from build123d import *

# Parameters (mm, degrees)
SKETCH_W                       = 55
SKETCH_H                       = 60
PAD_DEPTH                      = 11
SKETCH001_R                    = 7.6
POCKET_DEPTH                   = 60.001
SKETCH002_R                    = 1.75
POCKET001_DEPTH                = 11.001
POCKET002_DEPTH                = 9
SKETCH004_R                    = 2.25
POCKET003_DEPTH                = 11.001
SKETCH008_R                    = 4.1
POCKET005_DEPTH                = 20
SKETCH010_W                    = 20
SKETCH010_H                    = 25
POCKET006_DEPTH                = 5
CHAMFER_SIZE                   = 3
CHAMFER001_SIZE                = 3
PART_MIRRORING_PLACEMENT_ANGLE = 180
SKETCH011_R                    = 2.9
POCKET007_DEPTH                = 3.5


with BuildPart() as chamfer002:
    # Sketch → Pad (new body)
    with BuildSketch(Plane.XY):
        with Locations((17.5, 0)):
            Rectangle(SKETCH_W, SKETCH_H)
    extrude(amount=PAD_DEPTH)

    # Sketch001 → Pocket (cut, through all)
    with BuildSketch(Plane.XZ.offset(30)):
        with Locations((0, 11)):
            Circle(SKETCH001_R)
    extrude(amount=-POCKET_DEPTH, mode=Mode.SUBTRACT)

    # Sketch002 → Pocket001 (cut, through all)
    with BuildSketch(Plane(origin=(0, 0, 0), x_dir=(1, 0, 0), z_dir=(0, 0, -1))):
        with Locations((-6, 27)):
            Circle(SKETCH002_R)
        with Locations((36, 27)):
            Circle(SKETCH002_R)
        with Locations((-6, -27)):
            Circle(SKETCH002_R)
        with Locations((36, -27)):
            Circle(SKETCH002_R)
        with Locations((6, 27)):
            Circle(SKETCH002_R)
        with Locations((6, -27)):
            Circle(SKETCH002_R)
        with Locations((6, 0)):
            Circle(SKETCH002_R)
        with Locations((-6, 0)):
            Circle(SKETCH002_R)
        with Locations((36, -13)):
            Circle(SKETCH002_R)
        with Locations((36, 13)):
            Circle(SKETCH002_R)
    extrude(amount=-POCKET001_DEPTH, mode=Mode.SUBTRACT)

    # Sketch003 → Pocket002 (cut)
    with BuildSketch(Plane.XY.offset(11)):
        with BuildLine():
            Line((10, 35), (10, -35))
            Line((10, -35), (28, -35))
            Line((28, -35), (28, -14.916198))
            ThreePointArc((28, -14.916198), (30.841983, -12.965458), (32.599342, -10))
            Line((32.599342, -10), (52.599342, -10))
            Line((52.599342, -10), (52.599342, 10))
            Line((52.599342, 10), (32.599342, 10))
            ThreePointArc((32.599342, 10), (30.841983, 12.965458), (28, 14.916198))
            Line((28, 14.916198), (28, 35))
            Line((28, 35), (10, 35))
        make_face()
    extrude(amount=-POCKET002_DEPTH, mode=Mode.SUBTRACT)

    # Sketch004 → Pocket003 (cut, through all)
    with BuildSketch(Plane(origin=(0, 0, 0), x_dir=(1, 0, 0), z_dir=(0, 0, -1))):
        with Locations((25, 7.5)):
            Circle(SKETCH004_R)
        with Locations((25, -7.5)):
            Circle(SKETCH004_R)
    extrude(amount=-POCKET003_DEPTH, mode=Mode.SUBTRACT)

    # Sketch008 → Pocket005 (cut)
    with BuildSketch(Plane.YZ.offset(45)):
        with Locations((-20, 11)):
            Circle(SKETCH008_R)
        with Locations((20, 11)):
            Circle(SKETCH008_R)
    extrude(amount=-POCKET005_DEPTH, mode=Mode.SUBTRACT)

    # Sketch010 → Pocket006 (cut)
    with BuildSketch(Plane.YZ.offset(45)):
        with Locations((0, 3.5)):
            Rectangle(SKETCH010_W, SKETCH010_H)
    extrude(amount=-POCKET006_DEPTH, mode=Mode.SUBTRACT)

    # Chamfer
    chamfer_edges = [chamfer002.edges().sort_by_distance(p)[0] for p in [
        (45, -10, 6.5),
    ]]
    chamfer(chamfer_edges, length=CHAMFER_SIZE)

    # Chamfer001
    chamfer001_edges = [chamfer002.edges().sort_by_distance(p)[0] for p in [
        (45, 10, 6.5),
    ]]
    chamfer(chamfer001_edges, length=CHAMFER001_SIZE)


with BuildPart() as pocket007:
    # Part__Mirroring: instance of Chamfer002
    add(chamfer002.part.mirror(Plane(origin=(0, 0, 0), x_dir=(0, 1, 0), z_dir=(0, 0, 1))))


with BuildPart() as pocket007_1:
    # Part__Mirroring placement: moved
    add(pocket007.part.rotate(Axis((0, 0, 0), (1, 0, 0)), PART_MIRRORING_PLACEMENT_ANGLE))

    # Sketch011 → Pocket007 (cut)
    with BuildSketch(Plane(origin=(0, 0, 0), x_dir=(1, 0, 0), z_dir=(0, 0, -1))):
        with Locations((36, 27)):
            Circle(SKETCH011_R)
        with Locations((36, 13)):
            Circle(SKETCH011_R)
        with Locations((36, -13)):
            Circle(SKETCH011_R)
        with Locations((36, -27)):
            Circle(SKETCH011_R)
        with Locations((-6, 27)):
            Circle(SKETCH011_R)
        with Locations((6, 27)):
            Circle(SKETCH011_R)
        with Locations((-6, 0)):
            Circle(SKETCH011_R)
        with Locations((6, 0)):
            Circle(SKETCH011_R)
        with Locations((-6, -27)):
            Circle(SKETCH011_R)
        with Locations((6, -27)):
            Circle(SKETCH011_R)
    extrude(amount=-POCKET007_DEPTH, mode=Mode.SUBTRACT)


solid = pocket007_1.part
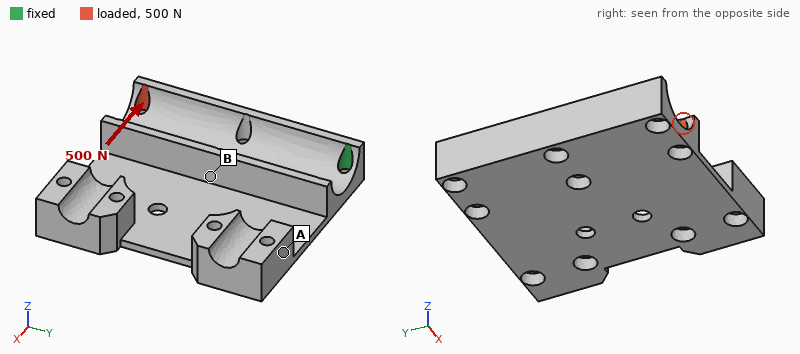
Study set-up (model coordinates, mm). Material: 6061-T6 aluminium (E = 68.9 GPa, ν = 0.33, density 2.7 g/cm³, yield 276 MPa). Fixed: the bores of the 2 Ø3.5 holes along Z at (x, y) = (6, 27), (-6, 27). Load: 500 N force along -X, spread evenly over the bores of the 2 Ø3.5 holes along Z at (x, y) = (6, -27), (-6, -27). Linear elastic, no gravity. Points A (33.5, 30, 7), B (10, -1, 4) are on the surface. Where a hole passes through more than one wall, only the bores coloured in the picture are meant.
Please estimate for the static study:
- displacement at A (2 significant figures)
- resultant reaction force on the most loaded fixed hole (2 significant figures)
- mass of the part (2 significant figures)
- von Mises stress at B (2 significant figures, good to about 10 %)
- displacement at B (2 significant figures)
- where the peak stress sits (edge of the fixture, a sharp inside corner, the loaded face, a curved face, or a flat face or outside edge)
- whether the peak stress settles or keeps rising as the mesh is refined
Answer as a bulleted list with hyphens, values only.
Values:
- 0.076 mm
- 1.7 kN
- 41 g
- 29 MPa
- 0.068 mm
- edge of the fixture
- keeps rising
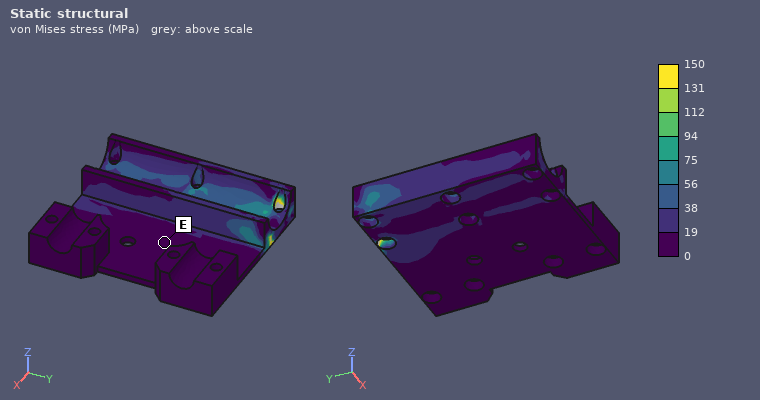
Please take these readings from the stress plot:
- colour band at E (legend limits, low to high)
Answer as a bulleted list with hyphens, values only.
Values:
- 0 to 19 MPa
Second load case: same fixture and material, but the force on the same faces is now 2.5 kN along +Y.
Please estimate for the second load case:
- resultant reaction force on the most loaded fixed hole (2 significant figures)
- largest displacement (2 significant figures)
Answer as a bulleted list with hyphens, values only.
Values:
- 1.3 kN
- 0.11 mm
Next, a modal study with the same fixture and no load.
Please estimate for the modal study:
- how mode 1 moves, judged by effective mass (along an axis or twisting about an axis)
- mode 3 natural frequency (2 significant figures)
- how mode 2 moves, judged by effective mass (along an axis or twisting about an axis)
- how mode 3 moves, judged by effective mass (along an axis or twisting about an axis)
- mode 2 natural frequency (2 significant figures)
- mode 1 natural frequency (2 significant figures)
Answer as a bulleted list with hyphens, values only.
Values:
- along Z
- 2000 Hz
- twisting about X
- along Z
- 1100 Hz
- 620 Hz
